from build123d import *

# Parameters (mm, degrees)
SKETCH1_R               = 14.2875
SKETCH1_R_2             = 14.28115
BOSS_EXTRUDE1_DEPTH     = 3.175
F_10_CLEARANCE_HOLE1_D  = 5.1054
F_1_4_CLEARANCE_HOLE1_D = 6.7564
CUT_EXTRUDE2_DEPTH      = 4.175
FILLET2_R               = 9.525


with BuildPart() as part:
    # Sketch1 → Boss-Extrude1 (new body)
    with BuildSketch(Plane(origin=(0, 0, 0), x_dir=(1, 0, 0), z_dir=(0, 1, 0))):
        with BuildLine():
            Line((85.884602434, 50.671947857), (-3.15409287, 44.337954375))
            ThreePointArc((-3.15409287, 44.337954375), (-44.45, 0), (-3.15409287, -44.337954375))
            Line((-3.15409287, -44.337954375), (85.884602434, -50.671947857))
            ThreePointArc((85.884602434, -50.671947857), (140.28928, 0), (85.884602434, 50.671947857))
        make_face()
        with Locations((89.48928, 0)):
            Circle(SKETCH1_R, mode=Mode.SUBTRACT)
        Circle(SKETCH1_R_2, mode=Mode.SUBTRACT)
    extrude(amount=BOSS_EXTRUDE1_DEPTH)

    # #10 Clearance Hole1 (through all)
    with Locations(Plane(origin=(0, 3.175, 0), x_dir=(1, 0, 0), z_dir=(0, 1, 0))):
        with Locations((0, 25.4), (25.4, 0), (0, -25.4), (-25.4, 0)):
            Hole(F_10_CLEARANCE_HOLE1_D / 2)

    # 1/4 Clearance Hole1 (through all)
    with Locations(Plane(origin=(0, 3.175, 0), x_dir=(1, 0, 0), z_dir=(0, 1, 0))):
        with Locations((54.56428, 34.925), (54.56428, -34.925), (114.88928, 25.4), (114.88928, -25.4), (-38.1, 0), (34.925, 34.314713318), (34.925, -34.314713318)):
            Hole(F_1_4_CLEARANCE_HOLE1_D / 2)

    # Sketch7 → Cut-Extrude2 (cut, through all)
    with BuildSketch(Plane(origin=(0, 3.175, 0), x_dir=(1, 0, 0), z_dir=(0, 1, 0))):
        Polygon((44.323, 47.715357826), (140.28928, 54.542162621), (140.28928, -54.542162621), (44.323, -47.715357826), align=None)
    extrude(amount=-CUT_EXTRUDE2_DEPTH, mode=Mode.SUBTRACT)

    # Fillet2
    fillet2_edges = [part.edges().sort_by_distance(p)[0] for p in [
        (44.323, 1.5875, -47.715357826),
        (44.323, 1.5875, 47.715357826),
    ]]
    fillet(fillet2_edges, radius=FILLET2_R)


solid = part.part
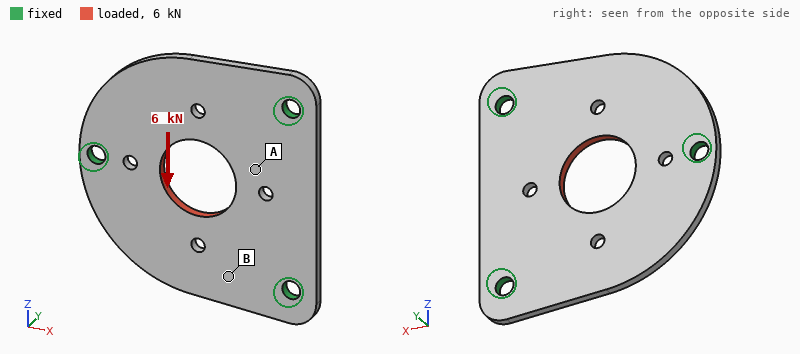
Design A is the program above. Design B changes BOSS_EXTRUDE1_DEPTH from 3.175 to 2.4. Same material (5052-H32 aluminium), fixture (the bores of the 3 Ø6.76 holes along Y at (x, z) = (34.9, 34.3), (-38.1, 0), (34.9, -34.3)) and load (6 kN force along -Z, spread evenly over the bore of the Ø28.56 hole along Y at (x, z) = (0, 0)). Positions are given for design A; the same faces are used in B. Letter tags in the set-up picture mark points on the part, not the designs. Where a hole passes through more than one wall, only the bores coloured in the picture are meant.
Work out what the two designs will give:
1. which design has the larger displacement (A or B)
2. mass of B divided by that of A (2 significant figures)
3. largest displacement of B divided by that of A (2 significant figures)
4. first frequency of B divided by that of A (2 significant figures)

B
0.76
1.3
0.77
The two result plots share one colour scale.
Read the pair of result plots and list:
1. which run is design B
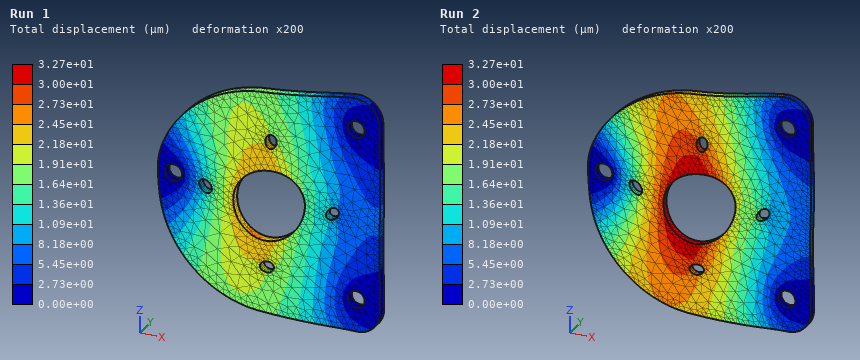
Run 2
